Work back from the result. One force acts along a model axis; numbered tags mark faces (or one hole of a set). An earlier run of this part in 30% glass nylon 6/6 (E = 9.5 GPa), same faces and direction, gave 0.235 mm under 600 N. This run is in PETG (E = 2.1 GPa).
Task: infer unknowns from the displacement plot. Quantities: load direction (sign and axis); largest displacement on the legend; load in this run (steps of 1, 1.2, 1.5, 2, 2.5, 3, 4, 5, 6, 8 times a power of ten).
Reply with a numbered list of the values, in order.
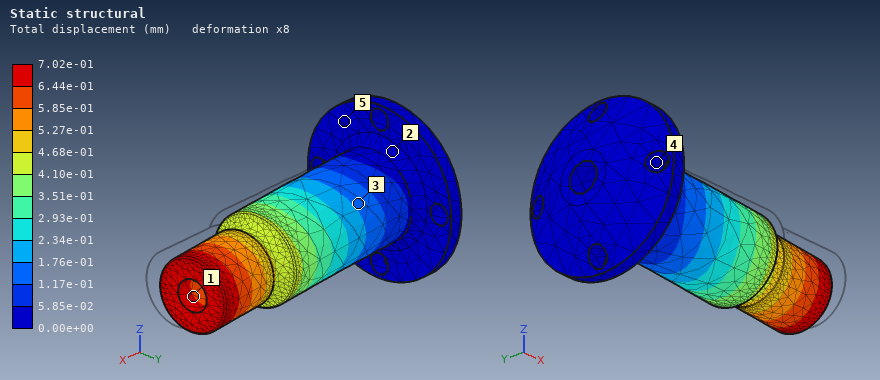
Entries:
1. +Y
2. 7.02e-01 mm
3. 400 N
